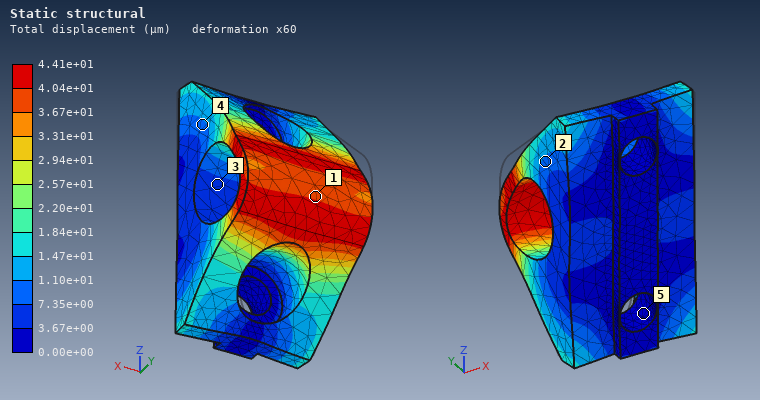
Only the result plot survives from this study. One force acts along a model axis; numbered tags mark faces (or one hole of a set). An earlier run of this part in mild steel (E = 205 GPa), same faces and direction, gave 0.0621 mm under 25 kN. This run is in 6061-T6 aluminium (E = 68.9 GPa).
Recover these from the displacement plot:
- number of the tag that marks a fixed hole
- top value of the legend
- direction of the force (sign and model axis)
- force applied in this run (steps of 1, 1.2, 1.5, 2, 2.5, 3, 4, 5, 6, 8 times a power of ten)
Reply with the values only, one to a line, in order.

5
4.41e+01 µm
-Z
6 kN
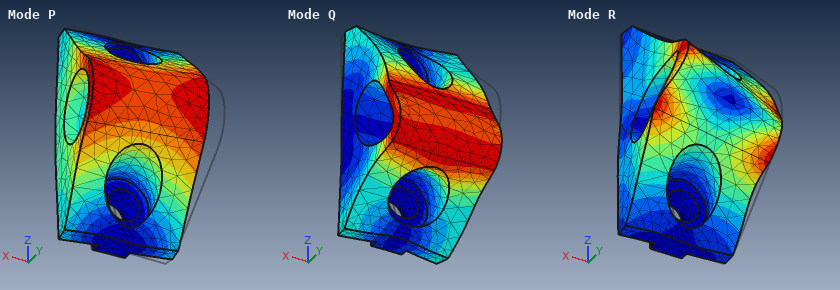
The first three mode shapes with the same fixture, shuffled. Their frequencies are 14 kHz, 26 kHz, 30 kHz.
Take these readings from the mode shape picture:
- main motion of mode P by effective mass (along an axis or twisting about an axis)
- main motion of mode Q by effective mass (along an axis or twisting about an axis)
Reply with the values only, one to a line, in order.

along X
along Z
